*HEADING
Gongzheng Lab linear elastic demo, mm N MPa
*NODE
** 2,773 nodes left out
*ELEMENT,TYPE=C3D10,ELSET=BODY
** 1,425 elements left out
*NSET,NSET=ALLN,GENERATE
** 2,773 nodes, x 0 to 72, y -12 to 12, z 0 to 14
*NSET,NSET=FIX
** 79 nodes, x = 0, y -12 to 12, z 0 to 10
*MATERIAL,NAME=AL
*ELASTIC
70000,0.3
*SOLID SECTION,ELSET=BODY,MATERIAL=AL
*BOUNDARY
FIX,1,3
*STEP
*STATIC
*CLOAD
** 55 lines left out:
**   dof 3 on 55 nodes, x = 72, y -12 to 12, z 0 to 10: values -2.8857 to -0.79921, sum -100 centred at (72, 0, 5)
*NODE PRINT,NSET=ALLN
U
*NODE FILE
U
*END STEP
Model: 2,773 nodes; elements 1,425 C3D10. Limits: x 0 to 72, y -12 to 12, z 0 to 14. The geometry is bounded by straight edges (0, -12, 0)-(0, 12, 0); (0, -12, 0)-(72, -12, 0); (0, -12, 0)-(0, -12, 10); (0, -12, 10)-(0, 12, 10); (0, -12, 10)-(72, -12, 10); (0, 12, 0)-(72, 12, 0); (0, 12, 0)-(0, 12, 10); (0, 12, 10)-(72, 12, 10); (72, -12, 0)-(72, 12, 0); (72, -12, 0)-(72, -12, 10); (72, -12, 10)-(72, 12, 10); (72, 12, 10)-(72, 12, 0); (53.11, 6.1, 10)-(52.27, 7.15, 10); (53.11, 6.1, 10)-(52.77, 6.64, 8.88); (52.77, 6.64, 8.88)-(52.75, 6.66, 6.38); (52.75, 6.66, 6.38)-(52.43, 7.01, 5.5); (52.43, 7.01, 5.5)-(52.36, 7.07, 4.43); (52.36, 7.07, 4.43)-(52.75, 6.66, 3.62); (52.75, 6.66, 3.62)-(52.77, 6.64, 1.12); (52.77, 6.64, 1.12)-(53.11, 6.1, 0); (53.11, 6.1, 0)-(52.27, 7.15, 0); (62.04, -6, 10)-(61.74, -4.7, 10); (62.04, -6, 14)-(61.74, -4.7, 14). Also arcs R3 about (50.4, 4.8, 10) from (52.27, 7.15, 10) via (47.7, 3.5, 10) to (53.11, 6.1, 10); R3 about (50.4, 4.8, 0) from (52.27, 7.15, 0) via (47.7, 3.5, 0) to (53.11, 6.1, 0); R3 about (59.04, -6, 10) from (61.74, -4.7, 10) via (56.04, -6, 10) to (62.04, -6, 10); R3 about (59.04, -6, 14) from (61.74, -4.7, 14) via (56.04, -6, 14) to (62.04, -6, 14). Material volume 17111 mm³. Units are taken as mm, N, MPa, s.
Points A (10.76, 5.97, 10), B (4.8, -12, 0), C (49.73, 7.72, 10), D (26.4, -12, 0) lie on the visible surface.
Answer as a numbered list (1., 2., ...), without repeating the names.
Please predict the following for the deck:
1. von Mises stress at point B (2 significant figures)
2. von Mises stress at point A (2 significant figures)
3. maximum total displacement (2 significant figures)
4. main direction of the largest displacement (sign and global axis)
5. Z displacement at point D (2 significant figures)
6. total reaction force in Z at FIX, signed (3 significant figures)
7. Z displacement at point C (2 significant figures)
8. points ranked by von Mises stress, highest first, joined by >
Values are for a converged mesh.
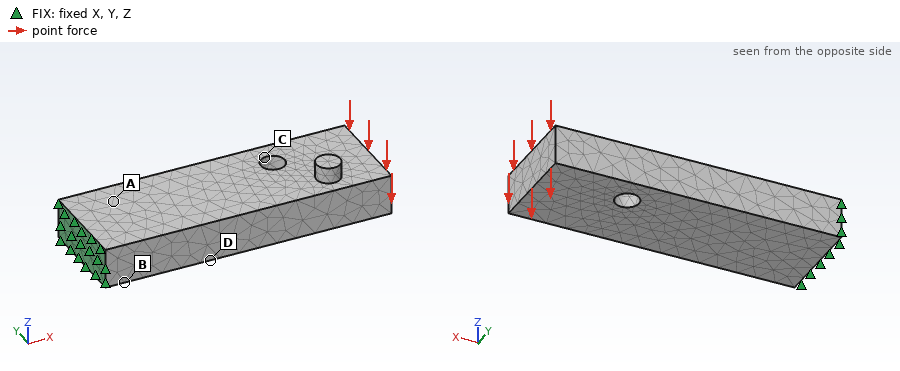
1. 16 MPa
2. 15 MPa
3. 0.090 mm
4. -Z
5. -0.015 mm
6. 100 N
7. -0.049 mm
8. B > A > C > D
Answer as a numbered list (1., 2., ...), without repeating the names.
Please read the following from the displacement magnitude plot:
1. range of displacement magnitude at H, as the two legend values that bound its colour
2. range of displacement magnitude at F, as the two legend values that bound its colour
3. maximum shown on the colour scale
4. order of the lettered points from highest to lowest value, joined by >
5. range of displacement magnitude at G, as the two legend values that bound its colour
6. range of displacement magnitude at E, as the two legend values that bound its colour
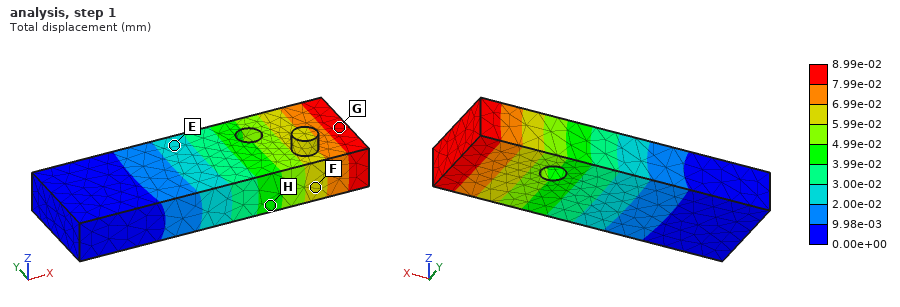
1. 3.99e-02 to 4.99e-02 mm
2. 5.99e-02 to 6.99e-02 mm
3. 8.99e-02 mm
4. G > F > H > E
5. 7.99e-02 to 8.99e-02 mm
6. 2.00e-02 to 3.00e-02 mm
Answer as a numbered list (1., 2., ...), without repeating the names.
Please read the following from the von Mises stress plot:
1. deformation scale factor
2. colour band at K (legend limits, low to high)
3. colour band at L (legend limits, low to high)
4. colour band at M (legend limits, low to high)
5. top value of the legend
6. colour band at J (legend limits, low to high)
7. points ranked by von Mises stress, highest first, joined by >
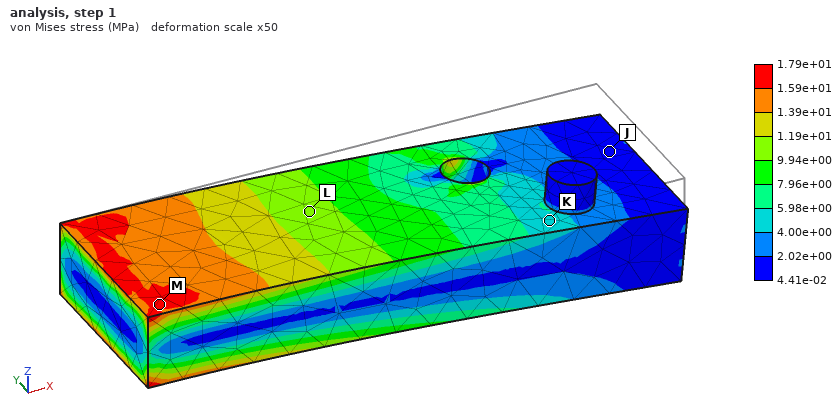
1. 50
2. 4.00e+00 to 5.98e+00 MPa
3. 9.94e+00 to 1.19e+01 MPa
4. 1.59e+01 to 1.79e+01 MPa
5. 1.79e+01 MPa
6. 4.41e-02 to 2.02e+00 MPa
7. M > L > K > J
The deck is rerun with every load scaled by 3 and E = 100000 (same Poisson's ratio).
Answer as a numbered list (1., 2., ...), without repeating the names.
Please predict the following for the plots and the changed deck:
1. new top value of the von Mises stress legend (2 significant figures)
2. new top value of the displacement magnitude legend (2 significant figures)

1. 54 MPa
2. 0.19 mm
